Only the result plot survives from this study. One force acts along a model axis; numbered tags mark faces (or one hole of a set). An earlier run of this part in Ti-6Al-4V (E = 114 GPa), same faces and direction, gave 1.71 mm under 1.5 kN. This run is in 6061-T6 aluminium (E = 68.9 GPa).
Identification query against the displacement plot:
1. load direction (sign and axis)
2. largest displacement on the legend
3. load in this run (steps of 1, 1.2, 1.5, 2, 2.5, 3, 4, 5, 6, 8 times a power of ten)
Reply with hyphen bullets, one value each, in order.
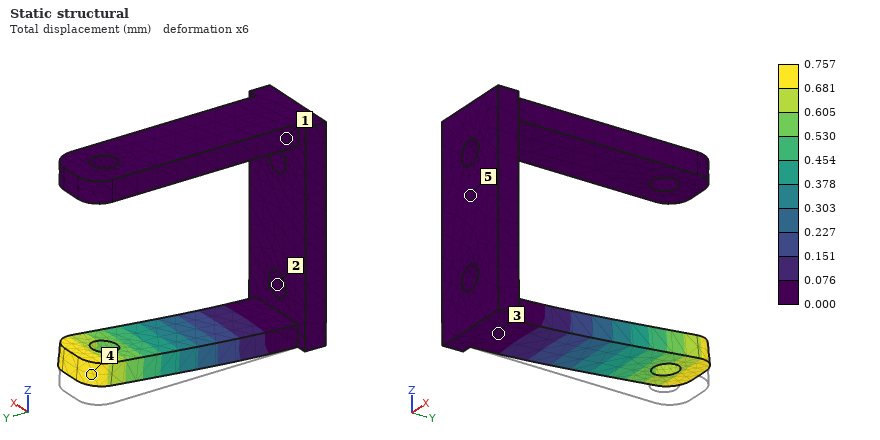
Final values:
- +Z
- 0.757 mm
- 400 N
